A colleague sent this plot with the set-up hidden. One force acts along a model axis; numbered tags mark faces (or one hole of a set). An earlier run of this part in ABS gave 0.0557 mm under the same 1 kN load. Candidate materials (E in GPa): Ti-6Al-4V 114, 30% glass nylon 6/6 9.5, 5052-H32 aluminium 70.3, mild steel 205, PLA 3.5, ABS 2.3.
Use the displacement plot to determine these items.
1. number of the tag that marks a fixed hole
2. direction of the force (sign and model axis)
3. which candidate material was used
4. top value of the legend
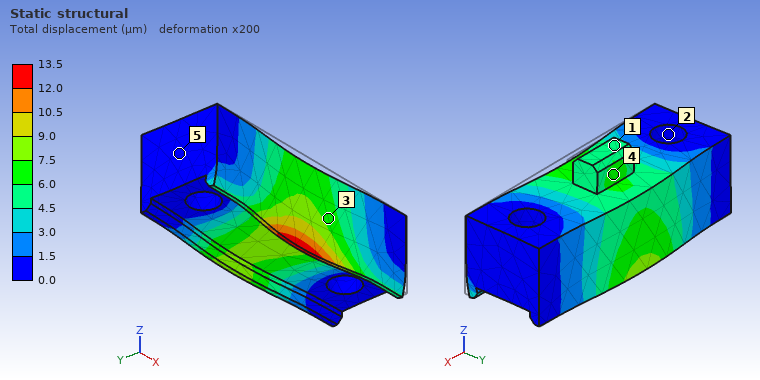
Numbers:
2
+Y
30% glass nylon 6/6
13.5 µm
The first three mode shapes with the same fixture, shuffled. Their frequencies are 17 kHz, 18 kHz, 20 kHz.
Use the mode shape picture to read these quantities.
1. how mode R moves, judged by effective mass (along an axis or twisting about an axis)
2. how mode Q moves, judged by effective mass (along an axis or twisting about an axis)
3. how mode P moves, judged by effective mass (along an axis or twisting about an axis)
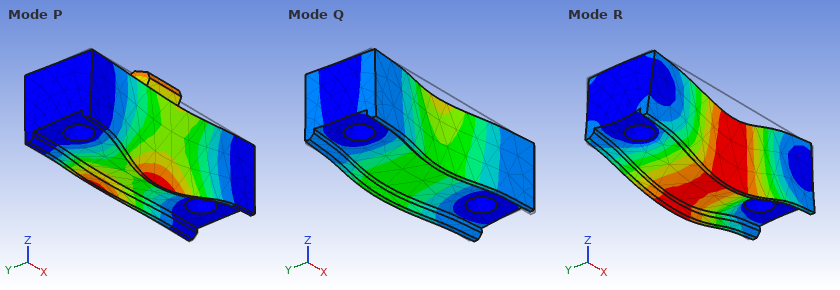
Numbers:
along Z
along Y
twisting about X
